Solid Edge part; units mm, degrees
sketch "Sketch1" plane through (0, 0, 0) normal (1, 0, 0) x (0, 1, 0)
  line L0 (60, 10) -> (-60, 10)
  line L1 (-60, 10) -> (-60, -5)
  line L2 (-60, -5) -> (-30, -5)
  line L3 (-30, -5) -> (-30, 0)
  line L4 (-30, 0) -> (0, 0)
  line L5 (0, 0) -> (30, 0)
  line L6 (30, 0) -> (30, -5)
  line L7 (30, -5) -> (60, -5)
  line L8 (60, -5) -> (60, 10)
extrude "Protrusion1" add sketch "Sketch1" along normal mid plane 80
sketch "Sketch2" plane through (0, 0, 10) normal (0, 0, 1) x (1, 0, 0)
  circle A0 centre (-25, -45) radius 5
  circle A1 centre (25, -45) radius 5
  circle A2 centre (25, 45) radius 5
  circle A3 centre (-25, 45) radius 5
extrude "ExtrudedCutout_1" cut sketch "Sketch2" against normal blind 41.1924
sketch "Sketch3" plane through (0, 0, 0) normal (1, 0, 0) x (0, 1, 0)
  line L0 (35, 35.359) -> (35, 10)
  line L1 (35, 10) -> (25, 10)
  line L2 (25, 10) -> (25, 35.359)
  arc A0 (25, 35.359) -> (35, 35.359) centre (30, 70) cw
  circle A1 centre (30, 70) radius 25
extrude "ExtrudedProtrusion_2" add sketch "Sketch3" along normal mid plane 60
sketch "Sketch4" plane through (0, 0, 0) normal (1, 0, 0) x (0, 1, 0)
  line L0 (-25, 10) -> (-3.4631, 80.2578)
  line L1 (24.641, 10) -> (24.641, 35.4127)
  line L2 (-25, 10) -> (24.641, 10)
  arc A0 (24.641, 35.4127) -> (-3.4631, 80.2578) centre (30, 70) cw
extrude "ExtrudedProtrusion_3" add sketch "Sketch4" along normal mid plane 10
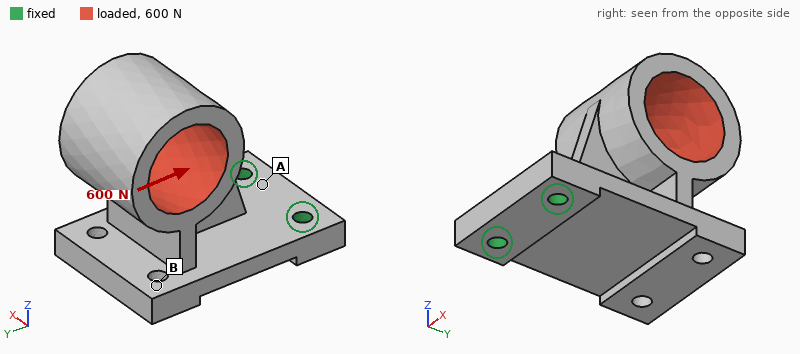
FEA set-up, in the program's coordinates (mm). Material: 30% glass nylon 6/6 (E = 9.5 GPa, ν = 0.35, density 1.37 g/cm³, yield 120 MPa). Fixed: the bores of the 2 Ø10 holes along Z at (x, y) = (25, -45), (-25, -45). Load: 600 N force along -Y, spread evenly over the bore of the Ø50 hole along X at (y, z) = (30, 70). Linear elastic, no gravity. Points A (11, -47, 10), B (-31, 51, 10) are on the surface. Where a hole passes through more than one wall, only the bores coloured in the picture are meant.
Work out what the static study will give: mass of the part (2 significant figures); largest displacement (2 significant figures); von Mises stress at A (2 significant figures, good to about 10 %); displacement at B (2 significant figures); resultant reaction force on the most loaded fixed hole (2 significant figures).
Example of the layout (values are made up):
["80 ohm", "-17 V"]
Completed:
["360 g", "1.9 mm", "5.0 MPa", "1.2 mm", "330 N"]
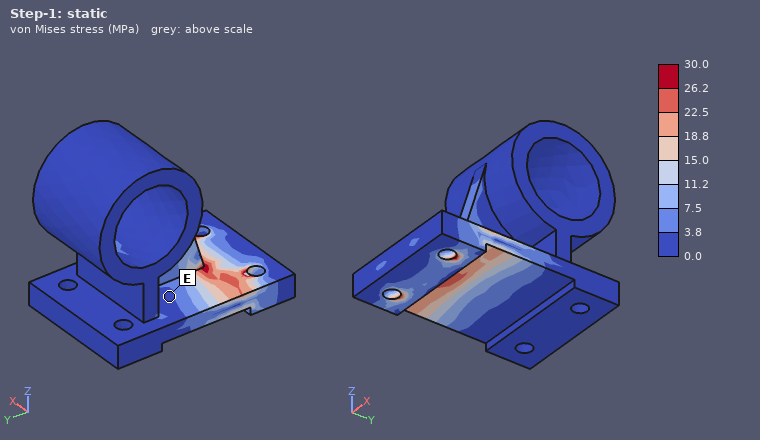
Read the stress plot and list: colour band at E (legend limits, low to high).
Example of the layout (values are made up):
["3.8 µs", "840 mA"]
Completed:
["0.0 to 3.8 MPa"]
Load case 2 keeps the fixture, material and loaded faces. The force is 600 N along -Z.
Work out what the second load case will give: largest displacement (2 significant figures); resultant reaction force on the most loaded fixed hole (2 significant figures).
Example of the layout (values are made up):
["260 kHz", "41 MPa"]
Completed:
["1.6 mm", "300 N"]
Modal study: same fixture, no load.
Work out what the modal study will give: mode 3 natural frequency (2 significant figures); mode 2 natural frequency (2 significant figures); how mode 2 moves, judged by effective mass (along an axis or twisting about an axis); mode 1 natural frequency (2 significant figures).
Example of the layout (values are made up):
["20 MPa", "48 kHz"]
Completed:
["1200 Hz", "310 Hz", "along X", "200 Hz"]
